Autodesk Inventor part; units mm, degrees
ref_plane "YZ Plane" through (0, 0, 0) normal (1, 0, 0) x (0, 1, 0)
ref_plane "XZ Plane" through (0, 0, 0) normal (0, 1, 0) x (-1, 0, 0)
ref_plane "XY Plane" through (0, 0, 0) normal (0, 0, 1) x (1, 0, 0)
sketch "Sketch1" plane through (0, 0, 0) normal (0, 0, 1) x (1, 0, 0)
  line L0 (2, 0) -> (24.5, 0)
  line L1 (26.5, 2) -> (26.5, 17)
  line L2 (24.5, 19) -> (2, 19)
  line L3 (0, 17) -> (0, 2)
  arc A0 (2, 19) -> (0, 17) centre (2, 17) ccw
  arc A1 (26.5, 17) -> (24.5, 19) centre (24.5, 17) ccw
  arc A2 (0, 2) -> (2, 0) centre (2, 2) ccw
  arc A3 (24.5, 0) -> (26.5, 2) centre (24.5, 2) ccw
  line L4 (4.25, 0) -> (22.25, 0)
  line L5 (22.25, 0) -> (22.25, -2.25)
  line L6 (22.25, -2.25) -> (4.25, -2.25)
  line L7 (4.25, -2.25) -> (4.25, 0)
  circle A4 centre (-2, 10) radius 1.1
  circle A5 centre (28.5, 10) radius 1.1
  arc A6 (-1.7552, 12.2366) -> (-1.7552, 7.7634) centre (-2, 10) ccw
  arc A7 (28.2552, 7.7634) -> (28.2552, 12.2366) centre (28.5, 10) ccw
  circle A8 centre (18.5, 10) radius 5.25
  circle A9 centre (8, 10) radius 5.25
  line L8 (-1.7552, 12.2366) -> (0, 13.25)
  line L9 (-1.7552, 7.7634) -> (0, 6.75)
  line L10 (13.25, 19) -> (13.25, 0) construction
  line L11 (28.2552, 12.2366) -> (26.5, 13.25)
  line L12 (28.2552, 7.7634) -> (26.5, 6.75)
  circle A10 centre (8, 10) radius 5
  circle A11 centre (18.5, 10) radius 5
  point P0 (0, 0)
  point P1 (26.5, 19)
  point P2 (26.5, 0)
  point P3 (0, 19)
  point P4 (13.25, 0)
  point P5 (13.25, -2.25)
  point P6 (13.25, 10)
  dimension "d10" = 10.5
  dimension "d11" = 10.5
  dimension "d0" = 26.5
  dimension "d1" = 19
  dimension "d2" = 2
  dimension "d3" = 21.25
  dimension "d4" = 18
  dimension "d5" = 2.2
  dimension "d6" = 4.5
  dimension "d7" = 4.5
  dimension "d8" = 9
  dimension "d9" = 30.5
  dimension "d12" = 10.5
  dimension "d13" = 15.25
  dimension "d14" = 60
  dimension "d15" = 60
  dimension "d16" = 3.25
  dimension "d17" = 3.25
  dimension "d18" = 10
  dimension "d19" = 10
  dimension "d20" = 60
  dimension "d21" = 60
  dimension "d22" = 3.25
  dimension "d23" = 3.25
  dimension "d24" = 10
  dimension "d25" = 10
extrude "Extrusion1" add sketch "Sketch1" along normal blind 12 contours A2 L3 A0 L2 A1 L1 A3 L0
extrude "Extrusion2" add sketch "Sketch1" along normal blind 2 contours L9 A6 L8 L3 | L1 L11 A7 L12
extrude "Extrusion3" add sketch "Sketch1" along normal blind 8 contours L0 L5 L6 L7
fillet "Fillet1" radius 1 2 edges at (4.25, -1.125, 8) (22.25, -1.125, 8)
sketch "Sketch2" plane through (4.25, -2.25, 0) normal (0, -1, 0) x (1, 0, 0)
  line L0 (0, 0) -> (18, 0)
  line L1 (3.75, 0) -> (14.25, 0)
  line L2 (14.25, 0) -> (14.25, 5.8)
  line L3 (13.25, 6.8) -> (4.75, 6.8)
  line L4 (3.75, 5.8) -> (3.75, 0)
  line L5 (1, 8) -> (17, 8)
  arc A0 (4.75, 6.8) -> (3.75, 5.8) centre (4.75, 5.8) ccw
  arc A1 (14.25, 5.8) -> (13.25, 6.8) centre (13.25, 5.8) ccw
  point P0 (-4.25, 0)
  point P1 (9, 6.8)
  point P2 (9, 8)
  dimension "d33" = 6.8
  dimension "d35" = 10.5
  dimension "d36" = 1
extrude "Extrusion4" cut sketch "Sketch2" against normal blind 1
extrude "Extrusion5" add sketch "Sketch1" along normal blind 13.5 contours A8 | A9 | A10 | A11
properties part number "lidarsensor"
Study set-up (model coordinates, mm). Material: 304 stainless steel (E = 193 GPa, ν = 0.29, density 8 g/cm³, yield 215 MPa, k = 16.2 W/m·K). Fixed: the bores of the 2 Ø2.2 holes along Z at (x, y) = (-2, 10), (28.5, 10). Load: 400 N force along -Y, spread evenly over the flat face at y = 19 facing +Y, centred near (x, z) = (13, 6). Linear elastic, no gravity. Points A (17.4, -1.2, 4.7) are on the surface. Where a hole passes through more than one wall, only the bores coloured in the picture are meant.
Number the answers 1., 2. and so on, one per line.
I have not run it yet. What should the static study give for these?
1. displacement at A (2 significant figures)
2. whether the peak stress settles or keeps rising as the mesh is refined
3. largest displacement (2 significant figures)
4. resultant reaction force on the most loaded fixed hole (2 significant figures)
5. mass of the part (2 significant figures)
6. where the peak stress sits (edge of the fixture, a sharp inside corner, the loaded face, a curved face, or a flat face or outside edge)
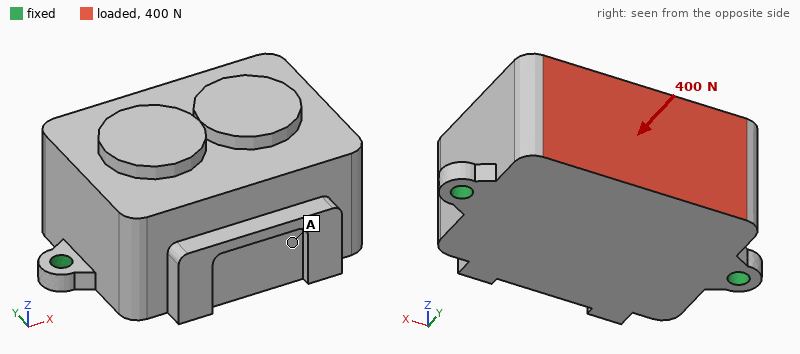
1. 21 µm
2. keeps rising
3. 27 µm
4. 200 N
5. 53 g
6. edge of the fixture
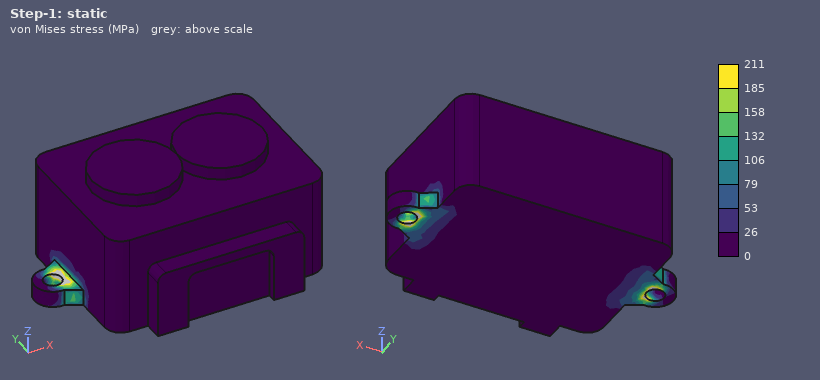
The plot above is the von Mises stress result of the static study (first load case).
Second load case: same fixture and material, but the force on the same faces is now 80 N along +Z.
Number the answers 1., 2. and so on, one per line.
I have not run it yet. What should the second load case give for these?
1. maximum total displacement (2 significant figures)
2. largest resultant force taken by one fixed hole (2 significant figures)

1. 9.3 µm
2. 46 N
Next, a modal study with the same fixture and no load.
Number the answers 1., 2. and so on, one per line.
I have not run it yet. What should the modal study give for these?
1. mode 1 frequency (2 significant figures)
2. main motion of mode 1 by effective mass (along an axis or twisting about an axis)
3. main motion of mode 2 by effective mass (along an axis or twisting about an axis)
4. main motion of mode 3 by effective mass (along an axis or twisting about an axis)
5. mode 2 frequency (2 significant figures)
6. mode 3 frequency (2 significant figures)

1. 2700 Hz
2. along Y
3. along Z
4. along X
5. 13 kHz
6. 18 kHz
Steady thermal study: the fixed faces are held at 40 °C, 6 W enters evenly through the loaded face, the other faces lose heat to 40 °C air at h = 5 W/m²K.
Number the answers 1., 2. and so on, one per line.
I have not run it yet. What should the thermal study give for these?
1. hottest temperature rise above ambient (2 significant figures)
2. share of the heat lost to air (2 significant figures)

1. 60 K
2. 8.2 %
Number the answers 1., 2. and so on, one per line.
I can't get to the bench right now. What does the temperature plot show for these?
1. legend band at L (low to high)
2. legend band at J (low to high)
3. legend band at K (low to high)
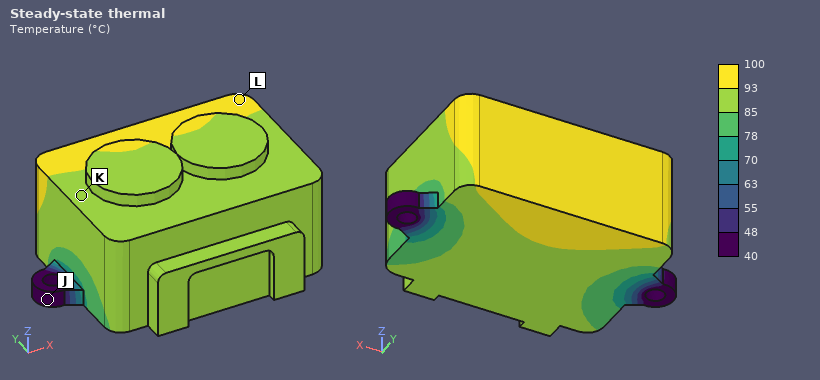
1. 93 to 100 °C
2. 40 to 48 °C
3. 85 to 93 °C
